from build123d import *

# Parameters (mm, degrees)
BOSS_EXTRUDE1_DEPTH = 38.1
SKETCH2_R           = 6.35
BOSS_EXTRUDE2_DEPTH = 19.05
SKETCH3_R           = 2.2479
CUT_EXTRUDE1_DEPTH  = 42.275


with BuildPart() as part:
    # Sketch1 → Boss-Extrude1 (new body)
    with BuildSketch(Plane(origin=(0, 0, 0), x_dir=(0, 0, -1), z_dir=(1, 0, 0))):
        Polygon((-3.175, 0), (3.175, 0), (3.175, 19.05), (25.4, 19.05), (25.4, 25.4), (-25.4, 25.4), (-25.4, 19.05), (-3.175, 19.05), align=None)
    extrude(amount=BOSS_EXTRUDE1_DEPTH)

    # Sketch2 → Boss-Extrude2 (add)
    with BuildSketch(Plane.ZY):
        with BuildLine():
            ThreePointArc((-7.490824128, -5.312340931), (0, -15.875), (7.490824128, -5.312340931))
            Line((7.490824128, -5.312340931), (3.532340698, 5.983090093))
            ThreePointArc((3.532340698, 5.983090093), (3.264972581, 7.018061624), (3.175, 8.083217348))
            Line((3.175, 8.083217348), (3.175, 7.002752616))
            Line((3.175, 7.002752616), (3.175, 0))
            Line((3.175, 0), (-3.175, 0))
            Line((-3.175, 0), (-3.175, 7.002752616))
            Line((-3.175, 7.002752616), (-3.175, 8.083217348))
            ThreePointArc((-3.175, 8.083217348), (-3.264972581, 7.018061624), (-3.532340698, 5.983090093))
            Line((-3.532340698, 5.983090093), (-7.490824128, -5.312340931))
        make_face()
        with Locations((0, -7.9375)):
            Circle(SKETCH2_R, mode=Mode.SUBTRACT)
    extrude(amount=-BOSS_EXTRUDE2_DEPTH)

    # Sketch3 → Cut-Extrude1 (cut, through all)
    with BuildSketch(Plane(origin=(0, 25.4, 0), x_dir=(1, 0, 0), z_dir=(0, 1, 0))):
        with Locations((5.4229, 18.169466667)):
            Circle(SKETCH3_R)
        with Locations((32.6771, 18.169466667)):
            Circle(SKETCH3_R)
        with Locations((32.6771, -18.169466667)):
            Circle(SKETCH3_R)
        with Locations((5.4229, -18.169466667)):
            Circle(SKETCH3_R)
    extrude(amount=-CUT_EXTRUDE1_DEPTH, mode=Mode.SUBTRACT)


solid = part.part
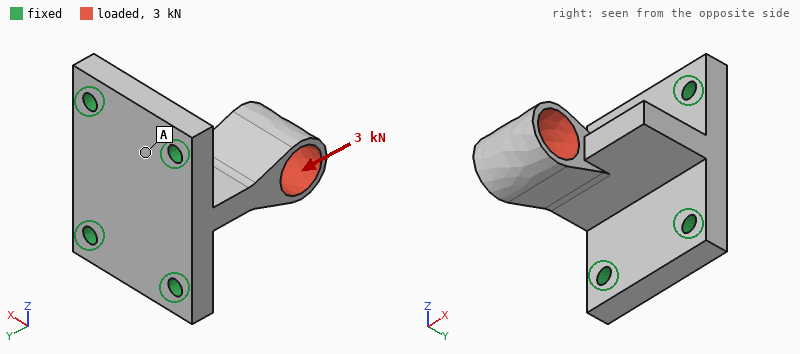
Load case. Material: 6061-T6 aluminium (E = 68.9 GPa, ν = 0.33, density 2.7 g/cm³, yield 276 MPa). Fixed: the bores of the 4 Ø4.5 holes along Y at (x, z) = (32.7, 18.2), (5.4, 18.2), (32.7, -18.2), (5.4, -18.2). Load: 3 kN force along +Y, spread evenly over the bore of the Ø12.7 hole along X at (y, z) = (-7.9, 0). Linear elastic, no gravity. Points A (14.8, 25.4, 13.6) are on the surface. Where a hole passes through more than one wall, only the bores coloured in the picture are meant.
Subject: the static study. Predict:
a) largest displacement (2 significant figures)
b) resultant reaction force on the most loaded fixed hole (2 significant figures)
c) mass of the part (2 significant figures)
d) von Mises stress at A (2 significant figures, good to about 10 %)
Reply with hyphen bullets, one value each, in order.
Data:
- 87 µm
- 1.3 kN
- 50 g
- 17 MPa
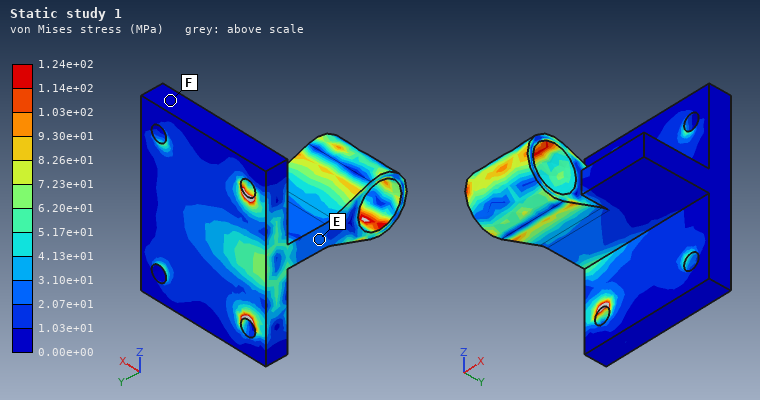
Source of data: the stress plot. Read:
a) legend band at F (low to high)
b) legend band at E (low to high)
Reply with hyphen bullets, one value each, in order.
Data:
- 0.00e+00 to 1.03e+01 MPa
- 2.07e+01 to 3.10e+01 MPa
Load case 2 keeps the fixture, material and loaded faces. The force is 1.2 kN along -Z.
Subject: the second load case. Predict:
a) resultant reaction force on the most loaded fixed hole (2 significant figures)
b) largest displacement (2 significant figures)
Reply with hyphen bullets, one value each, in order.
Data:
- 930 N
- 0.42 mm
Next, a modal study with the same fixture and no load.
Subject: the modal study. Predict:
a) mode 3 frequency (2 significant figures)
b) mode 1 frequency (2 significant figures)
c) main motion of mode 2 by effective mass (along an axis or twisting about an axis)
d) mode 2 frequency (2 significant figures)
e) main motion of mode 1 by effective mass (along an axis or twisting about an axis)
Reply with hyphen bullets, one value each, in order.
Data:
- 13 kHz
- 4500 Hz
- along X
- 8300 Hz
- along Z
